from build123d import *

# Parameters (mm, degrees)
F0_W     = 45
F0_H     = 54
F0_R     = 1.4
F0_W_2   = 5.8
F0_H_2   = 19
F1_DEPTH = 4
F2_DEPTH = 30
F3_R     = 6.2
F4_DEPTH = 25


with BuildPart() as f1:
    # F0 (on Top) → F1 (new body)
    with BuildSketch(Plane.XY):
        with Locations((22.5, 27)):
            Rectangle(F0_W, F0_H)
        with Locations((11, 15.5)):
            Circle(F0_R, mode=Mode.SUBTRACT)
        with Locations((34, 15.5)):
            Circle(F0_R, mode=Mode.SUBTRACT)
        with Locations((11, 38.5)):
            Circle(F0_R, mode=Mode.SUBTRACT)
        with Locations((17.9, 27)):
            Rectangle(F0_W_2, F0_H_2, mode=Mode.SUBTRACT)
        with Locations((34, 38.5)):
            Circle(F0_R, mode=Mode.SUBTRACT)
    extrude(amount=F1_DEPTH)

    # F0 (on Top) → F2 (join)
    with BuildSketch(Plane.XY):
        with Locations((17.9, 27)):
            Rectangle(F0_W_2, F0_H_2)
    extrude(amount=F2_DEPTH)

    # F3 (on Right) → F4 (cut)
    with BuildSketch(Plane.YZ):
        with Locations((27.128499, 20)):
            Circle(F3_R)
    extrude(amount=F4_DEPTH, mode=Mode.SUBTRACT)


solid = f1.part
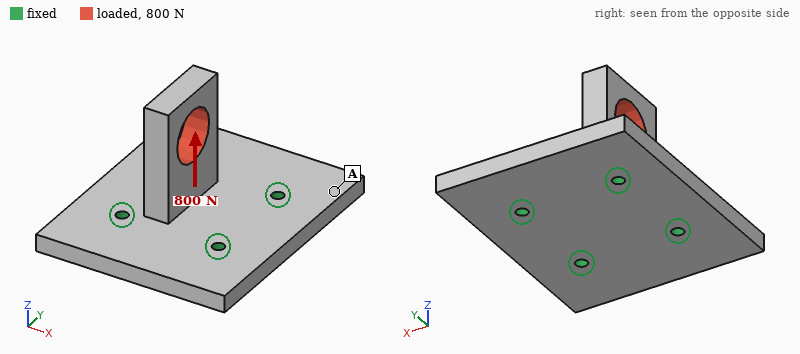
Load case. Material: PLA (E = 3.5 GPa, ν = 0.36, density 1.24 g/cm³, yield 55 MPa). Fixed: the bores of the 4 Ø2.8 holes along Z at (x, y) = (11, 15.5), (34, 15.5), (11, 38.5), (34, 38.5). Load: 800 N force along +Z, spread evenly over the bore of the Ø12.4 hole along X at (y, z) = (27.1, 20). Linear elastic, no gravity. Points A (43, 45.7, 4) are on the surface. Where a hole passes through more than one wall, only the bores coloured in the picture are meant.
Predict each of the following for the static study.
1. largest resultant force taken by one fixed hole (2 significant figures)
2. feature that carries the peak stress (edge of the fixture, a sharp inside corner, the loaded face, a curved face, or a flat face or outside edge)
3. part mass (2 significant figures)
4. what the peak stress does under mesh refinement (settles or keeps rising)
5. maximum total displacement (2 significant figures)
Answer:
300 N
edge of the fixture
15 g
keeps rising
0.27 mm
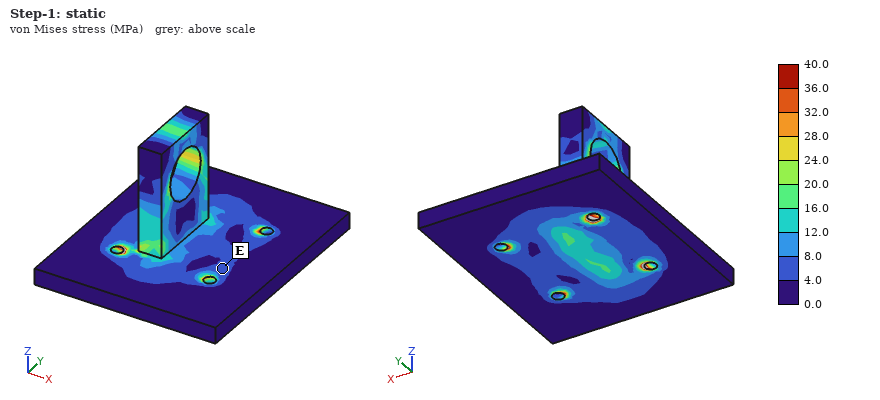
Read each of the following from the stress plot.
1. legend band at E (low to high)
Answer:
4.0 to 8.0 MPa
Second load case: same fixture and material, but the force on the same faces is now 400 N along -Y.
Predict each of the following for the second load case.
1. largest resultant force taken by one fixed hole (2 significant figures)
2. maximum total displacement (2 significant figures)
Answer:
300 N
0.57 mm
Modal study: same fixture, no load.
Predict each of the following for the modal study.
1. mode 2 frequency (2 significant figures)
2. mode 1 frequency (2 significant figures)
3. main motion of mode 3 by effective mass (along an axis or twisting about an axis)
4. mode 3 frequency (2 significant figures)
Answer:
3500 Hz
1900 Hz
along Z
3800 Hz
